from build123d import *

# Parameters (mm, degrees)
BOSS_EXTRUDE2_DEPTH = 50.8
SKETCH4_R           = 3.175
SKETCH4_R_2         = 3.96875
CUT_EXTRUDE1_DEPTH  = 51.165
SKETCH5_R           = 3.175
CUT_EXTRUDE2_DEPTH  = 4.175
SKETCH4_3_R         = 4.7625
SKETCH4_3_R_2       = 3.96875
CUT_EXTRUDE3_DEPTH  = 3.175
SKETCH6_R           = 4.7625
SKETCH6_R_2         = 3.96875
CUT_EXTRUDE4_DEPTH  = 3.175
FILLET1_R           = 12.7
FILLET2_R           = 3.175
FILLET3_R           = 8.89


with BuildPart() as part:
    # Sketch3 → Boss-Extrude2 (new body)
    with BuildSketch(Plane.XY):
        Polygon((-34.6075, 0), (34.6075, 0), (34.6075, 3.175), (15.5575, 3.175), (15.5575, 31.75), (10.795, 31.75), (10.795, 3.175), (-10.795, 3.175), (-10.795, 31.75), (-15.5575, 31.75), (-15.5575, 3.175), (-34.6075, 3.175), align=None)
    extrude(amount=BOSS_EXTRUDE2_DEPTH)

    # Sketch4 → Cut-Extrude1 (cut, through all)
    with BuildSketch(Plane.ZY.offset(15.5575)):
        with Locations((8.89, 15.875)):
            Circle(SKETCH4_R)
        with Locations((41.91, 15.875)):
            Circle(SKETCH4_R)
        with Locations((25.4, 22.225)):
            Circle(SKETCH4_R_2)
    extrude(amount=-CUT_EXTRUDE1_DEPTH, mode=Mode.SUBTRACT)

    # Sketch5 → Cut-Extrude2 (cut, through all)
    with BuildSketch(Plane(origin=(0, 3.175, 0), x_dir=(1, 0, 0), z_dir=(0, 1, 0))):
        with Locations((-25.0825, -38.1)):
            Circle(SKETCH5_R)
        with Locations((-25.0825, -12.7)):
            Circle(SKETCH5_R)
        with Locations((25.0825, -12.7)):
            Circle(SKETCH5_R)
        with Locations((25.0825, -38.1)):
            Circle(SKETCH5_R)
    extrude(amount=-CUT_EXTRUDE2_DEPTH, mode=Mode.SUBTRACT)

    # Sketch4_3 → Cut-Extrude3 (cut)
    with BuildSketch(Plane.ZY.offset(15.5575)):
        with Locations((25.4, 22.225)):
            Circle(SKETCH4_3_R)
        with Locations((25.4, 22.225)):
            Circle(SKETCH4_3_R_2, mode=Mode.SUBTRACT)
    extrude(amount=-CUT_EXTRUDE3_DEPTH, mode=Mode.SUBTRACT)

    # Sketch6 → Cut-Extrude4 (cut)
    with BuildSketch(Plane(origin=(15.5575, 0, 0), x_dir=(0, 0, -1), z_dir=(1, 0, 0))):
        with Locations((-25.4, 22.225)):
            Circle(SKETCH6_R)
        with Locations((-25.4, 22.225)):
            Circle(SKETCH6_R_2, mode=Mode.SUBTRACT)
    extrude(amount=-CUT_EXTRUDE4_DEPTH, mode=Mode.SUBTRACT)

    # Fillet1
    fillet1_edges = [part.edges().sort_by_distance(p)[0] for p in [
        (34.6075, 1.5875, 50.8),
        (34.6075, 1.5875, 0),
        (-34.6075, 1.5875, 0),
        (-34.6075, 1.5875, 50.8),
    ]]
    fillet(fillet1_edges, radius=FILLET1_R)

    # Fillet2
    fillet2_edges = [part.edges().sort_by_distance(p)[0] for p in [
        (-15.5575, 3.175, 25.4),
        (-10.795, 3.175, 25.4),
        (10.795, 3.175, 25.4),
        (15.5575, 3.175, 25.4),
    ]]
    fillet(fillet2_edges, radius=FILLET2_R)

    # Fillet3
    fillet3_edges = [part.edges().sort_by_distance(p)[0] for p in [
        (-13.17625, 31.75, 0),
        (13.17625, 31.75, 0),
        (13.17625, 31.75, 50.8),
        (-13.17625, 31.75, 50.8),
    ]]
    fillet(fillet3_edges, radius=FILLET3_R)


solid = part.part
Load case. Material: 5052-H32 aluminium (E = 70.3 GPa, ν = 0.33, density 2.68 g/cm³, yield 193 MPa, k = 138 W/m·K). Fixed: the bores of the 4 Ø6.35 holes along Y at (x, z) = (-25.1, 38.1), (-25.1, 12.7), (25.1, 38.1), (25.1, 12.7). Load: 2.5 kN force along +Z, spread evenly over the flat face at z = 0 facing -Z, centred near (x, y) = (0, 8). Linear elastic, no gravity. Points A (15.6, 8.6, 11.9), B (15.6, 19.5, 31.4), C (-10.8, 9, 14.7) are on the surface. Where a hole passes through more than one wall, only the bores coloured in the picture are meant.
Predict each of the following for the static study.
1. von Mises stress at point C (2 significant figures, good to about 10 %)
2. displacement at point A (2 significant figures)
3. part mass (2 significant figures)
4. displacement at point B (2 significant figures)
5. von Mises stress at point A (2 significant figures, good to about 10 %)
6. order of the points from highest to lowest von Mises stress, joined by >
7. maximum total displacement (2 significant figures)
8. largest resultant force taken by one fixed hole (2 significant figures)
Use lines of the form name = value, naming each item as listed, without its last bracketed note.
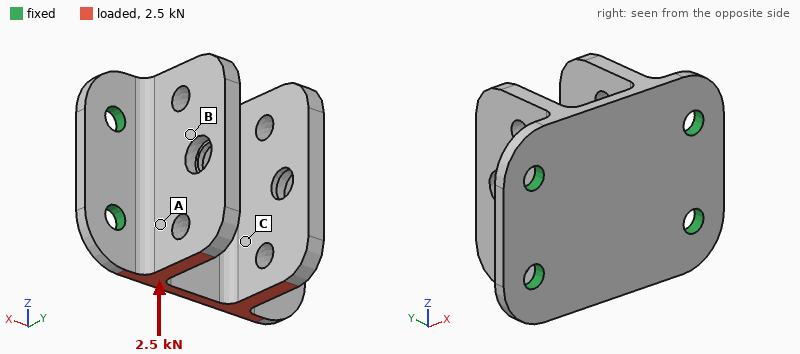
von Mises stress at point C = 10 MPa
displacement at point A = 12 µm
part mass = 62 g
displacement at point B = 16 µm
von Mises stress at point A = 17 MPa
order of the points from highest to lowest von Mises stress, joined by > = A > C > B
maximum total displacement = 29 µm
largest resultant force taken by one fixed hole = 780 N
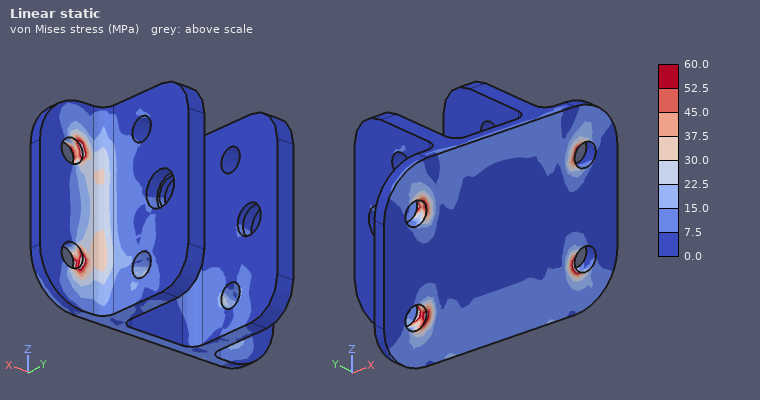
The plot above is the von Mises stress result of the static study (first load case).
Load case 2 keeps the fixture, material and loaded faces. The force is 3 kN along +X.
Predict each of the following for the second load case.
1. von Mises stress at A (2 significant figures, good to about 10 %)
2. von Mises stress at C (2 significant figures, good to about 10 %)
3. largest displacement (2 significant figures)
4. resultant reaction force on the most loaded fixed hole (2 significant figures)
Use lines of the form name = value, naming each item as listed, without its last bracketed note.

von Mises stress at A = 47 MPa
von Mises stress at C = 40 MPa
largest displacement = 0.13 mm
resultant reaction force on the most loaded fixed hole = 1.6 kN
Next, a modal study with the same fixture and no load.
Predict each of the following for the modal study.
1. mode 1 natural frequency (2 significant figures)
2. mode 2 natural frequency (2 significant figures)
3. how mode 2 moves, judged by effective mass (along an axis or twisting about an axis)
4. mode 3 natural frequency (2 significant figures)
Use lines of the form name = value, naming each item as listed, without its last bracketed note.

mode 1 natural frequency = 2600 Hz
mode 2 natural frequency = 4200 Hz
how mode 2 moves, judged by effective mass = along X
mode 3 natural frequency = 4700 Hz
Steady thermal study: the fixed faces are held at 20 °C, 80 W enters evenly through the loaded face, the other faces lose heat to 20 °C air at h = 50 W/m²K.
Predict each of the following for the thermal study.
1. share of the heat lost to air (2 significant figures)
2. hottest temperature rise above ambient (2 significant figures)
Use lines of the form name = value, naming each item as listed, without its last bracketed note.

share of the heat lost to air = 13 %
hottest temperature rise above ambient = 45 K
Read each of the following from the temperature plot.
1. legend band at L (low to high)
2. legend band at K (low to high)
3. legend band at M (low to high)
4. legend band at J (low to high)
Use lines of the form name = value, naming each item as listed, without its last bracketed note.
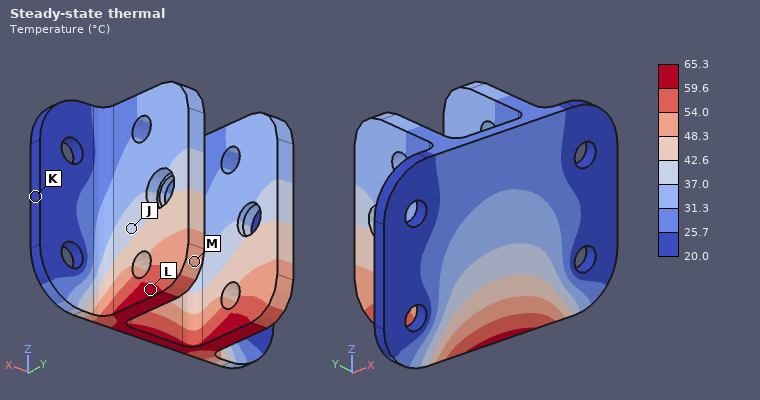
legend band at L = 59.6 to 65.3 °C
legend band at K = 20.0 to 25.7 °C
legend band at M = 48.3 to 54.0 °C
legend band at J = 37.0 to 42.6 °C
